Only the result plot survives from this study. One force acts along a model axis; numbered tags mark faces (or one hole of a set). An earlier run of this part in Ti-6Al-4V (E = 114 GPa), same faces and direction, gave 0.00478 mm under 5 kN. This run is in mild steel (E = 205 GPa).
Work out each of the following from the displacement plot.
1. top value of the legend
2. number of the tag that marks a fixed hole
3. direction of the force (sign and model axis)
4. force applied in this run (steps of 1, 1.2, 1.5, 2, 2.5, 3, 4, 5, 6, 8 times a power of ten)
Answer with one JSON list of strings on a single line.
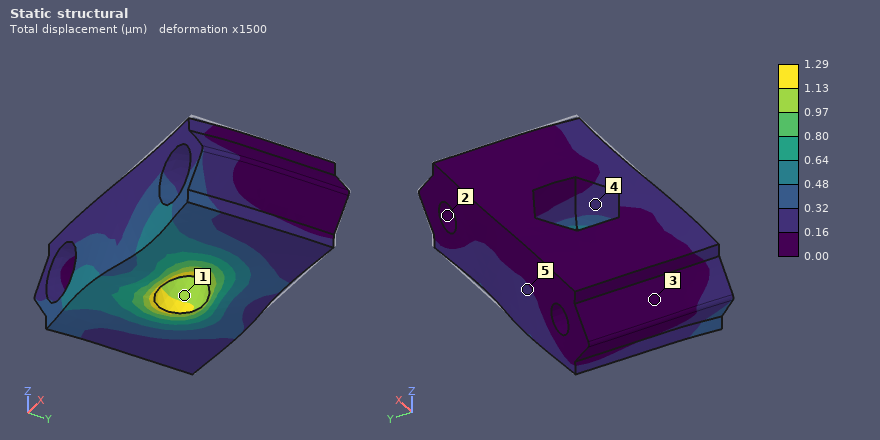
["1.29 µm", "2", "-X", "2.5 kN"]
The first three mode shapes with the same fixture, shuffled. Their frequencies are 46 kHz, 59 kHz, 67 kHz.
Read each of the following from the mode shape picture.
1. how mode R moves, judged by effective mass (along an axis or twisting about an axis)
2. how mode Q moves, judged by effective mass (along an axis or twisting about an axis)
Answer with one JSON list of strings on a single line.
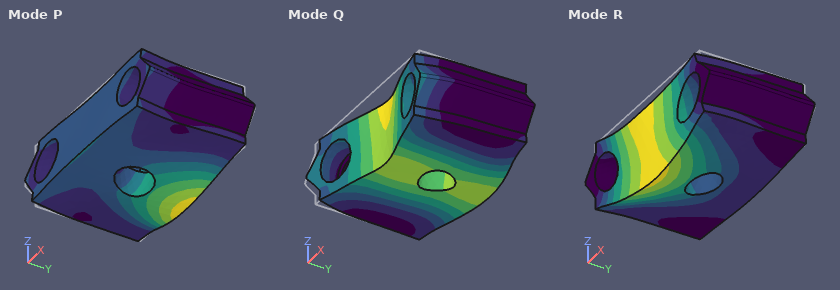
["along Z", "along Y"]
